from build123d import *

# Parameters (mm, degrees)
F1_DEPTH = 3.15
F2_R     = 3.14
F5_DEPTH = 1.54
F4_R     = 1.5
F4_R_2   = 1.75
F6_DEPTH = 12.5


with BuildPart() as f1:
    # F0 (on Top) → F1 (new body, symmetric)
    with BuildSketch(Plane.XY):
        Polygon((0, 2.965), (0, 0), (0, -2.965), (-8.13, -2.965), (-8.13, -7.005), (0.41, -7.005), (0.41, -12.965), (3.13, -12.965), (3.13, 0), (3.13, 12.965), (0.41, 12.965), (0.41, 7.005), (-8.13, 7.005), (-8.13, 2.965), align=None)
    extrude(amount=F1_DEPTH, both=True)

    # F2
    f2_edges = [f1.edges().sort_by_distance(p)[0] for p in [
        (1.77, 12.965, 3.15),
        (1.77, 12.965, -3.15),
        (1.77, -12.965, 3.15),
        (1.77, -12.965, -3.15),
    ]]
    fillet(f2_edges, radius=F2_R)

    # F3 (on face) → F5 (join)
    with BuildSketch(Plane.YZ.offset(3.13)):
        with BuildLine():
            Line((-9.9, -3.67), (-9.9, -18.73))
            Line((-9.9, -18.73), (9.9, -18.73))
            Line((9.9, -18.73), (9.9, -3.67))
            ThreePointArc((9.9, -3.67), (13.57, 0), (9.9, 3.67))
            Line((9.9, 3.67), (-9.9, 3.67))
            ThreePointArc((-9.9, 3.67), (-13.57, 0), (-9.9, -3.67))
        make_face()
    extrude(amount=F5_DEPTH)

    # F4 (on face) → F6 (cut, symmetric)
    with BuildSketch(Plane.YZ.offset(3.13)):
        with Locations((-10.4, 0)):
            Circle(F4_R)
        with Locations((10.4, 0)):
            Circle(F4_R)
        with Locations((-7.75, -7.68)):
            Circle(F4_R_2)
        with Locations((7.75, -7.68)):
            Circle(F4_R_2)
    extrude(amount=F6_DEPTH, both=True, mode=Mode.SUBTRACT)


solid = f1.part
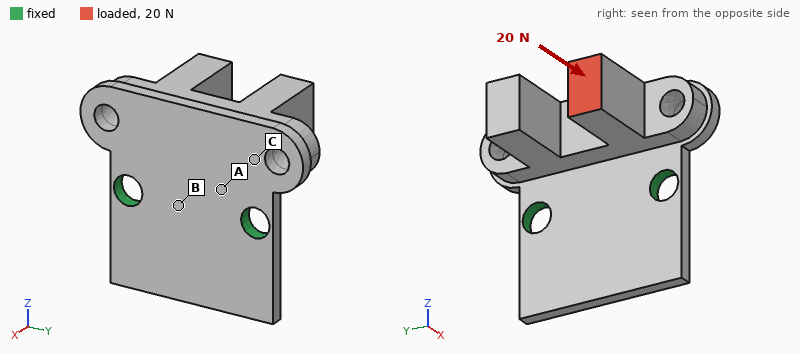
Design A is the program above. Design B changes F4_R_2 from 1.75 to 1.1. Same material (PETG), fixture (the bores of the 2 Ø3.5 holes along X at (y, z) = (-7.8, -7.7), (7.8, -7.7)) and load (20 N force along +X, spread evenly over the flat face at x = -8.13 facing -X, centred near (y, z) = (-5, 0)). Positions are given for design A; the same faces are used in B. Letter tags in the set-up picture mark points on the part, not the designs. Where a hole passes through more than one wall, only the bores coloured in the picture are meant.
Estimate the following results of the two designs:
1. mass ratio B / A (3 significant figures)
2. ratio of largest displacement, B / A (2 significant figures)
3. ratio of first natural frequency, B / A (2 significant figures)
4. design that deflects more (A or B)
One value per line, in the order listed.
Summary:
1.01
1.3
0.87
B
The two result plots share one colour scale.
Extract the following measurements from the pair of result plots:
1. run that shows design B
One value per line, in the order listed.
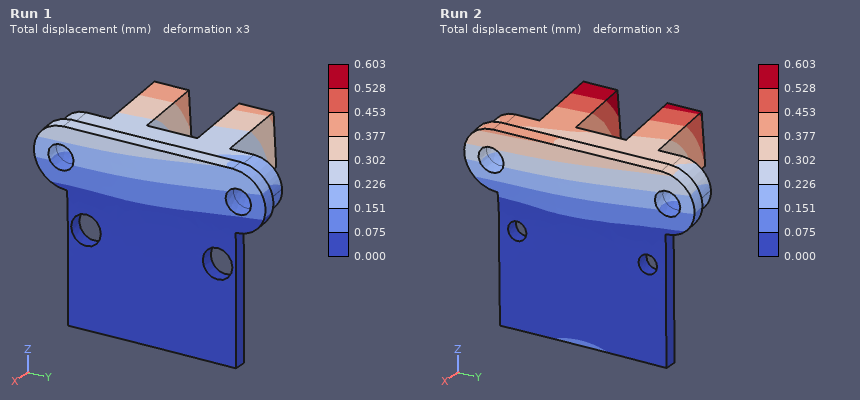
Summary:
Run 2
